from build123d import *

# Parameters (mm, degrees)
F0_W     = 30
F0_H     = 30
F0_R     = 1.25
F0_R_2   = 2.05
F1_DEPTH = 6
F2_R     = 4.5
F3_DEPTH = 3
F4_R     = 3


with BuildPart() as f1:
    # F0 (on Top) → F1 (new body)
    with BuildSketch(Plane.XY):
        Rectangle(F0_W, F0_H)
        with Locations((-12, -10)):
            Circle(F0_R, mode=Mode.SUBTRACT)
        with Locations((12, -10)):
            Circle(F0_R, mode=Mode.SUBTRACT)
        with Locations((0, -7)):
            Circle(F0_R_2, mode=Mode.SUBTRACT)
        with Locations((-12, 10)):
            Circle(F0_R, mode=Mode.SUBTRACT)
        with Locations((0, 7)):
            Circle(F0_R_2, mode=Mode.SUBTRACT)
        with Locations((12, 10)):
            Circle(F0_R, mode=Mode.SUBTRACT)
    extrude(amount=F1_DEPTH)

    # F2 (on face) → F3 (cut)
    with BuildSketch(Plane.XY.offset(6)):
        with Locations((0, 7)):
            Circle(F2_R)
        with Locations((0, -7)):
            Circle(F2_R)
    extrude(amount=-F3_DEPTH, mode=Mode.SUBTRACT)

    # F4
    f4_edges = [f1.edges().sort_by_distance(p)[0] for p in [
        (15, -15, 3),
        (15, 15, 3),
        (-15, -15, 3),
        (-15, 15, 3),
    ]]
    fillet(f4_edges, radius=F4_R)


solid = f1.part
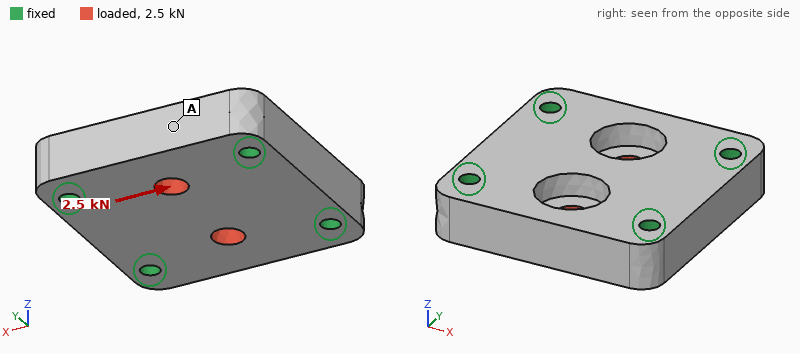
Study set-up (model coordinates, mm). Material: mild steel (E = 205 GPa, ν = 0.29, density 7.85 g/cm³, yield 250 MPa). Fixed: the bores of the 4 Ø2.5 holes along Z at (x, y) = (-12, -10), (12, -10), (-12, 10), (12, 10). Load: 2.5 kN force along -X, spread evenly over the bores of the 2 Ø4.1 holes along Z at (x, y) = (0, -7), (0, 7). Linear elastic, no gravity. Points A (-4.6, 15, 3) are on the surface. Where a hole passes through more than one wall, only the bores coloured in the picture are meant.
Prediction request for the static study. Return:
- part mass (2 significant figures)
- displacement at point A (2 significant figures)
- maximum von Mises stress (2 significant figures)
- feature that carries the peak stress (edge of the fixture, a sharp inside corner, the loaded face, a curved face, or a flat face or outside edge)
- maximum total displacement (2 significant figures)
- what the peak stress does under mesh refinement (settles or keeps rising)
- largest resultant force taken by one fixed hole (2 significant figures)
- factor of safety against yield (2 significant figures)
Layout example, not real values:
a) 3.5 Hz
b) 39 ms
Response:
a) 37 g
b) 0.30 µm
c) 55 MPa
d) the loaded face
e) 1.2 µm
f) settles
g) 650 N
h) 4.5
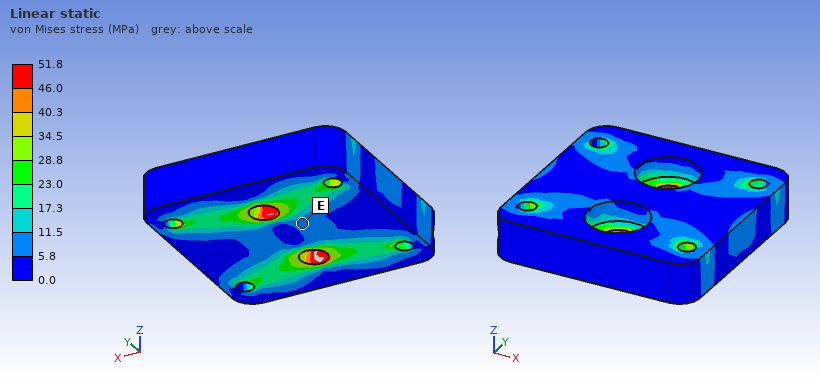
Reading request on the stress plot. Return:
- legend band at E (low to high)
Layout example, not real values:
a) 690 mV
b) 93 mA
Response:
a) 5.8 to 11.5 MPa
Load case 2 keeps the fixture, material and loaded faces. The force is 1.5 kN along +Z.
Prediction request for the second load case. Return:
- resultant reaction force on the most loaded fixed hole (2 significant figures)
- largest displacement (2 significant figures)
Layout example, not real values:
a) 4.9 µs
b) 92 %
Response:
a) 390 N
b) 4.3 µm
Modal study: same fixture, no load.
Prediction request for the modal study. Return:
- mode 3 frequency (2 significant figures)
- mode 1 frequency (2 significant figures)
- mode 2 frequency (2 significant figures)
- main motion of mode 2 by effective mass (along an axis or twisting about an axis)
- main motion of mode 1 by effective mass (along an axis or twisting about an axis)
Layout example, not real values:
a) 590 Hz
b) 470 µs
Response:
a) 48 kHz
b) 34 kHz
c) 44 kHz
d) twisting about X
e) along Z
